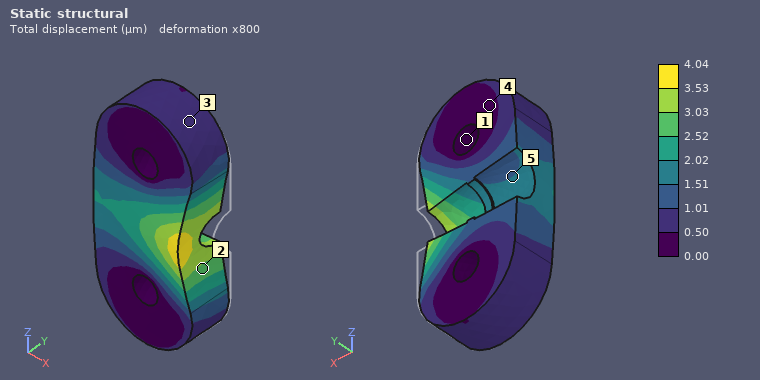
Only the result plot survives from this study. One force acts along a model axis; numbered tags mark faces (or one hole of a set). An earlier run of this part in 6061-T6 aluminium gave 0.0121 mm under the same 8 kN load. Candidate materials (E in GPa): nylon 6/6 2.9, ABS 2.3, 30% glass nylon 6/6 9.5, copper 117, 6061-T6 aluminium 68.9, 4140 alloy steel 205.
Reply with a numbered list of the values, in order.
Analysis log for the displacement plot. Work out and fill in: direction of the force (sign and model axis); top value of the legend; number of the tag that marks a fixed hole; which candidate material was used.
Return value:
1. -X
2. 4.04 µm
3. 1
4. 4140 alloy steel
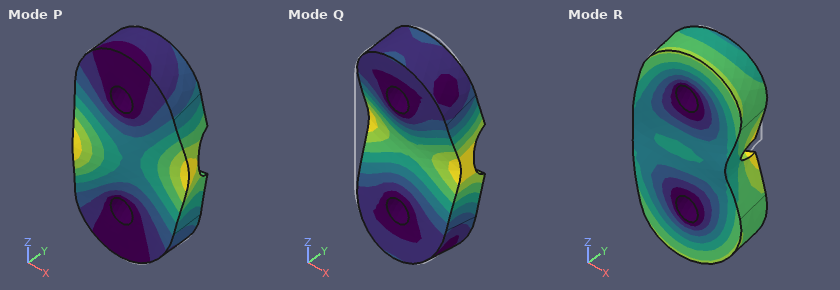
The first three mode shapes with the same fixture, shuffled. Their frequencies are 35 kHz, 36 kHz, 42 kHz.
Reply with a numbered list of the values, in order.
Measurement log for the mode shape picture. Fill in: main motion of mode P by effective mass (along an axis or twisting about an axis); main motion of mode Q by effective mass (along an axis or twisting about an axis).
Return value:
1. twisting about Z
2. along Y
